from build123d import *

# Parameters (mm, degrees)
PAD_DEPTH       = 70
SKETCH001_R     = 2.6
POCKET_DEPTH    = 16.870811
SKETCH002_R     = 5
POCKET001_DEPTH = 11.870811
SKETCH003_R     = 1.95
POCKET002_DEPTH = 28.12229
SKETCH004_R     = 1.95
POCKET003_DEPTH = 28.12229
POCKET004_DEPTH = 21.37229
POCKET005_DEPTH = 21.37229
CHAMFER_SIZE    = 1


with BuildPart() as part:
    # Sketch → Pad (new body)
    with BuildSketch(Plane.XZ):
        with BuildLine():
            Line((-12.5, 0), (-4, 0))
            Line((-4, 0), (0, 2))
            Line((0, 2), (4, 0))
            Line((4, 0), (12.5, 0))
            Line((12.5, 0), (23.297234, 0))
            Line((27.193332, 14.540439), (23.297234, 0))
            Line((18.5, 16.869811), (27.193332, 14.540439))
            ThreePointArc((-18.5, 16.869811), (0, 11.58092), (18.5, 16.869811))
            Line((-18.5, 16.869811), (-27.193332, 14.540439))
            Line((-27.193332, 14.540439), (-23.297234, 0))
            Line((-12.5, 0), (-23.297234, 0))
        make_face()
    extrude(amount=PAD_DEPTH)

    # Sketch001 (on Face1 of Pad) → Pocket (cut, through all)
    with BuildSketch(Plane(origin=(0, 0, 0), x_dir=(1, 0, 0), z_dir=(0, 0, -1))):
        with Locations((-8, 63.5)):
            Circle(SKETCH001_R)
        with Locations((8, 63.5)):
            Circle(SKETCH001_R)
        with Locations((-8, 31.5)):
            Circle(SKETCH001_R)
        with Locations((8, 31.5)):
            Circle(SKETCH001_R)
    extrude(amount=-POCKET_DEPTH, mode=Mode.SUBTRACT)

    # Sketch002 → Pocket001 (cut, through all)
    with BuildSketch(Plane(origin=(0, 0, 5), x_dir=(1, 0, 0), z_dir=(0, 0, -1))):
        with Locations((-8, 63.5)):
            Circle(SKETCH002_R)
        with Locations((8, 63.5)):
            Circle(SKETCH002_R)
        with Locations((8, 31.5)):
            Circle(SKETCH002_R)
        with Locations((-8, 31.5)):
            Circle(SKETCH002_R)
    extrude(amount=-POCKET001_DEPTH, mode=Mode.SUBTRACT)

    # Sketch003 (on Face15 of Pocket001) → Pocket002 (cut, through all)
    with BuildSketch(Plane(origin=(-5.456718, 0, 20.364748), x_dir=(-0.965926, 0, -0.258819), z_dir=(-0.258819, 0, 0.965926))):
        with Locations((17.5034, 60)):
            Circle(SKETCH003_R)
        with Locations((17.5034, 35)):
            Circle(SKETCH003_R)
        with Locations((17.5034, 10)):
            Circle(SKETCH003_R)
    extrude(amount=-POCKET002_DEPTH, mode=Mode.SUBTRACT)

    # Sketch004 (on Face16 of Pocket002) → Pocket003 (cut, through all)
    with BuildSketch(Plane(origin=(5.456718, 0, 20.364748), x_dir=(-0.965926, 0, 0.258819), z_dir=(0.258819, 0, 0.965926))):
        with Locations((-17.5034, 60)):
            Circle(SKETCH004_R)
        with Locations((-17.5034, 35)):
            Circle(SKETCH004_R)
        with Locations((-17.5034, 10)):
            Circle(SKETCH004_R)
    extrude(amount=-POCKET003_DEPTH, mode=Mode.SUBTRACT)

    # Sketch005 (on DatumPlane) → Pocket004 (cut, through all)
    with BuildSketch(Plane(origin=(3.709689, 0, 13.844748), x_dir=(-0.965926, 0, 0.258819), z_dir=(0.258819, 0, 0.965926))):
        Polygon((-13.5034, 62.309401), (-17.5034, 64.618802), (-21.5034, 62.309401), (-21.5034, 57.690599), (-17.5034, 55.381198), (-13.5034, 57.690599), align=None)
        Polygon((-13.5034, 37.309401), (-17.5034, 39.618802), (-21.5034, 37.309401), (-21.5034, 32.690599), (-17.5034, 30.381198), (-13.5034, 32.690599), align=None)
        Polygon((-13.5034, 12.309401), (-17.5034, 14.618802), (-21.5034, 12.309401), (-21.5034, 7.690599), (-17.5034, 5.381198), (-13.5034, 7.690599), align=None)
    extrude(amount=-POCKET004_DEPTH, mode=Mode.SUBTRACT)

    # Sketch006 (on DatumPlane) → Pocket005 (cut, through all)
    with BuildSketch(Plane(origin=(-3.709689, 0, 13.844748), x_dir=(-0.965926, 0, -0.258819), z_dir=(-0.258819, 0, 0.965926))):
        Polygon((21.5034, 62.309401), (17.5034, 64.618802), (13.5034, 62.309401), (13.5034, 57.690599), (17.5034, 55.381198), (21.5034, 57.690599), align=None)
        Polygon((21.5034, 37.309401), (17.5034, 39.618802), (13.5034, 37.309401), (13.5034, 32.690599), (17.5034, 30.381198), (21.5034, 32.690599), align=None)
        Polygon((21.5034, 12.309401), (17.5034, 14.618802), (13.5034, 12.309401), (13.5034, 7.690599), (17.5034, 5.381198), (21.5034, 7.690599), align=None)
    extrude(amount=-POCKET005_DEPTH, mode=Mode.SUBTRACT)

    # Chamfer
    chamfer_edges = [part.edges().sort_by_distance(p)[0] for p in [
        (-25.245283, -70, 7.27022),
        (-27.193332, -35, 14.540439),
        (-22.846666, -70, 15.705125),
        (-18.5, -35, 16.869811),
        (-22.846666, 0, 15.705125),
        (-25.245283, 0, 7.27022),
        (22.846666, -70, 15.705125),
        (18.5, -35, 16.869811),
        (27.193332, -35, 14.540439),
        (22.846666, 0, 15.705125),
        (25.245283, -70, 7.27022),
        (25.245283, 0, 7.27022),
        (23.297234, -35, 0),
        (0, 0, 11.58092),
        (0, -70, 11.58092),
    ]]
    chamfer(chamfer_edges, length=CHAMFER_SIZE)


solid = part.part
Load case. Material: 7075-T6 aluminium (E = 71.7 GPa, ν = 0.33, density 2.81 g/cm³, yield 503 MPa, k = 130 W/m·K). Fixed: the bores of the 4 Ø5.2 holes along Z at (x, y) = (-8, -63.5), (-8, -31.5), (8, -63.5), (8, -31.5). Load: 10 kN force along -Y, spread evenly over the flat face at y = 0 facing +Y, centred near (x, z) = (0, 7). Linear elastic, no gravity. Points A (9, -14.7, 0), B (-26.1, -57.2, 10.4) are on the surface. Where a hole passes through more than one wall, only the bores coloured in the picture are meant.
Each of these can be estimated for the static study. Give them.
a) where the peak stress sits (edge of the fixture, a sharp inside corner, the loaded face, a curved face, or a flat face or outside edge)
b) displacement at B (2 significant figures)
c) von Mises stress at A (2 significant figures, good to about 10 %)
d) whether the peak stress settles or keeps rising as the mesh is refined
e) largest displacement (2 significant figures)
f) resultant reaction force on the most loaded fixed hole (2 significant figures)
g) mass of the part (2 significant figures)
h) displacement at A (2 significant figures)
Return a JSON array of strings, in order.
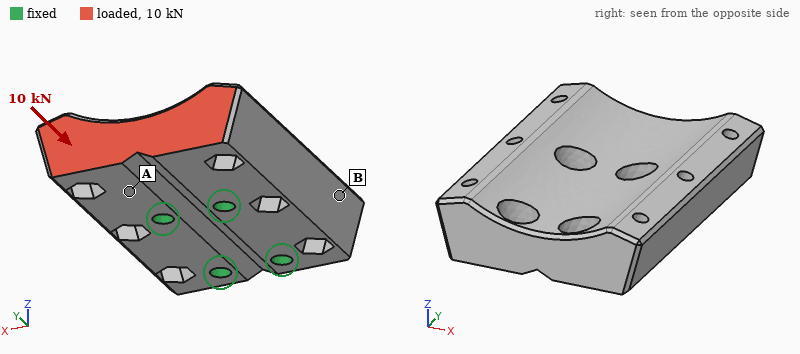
["edge of the fixture", "4.6 µm", "30 MPa", "keeps rising", "20 µm", "3.7 kN", "120 g", "9.7 µm"]
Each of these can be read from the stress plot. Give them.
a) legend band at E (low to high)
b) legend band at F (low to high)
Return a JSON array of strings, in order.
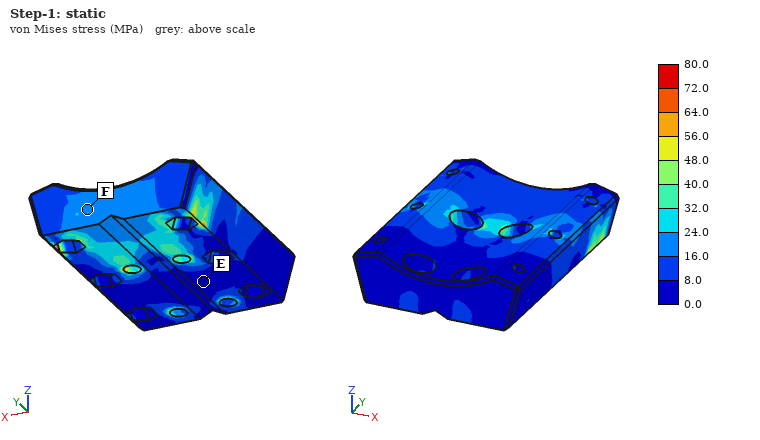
["0.0 to 8.0 MPa", "16.0 to 24.0 MPa"]
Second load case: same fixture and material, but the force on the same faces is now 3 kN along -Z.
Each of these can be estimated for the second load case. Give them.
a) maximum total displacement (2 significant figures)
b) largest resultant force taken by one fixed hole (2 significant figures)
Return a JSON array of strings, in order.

["97 µm", "3.2 kN"]
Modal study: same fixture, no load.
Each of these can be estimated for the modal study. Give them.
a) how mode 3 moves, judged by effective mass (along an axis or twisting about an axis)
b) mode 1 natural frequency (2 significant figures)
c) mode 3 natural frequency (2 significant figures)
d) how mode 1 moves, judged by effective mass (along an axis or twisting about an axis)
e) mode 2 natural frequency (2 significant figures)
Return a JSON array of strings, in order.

["along X", "6700 Hz", "12 kHz", "along Z", "8100 Hz"]
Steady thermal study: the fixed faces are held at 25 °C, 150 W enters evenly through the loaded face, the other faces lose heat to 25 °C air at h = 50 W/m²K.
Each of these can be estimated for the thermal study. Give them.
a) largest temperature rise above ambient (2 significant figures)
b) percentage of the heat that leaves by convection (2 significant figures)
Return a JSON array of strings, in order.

["77 K", "9.4 %"]
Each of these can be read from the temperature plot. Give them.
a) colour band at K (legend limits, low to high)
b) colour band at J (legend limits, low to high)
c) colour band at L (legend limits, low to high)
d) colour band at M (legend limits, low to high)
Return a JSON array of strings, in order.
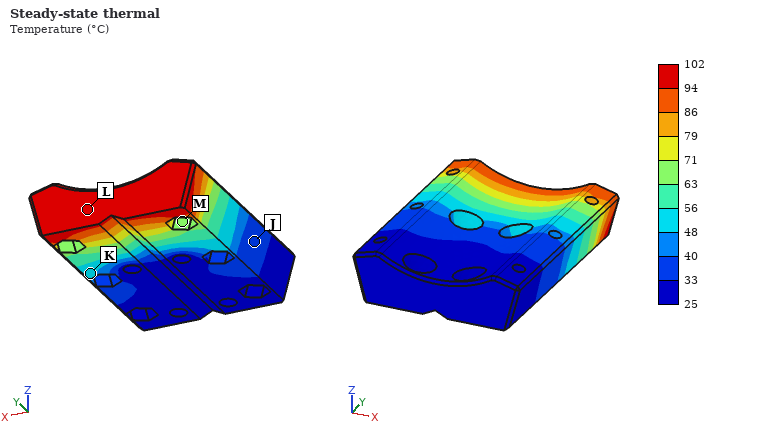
["48 to 56 °C", "33 to 40 °C", "94 to 102 °C", "63 to 71 °C"]
